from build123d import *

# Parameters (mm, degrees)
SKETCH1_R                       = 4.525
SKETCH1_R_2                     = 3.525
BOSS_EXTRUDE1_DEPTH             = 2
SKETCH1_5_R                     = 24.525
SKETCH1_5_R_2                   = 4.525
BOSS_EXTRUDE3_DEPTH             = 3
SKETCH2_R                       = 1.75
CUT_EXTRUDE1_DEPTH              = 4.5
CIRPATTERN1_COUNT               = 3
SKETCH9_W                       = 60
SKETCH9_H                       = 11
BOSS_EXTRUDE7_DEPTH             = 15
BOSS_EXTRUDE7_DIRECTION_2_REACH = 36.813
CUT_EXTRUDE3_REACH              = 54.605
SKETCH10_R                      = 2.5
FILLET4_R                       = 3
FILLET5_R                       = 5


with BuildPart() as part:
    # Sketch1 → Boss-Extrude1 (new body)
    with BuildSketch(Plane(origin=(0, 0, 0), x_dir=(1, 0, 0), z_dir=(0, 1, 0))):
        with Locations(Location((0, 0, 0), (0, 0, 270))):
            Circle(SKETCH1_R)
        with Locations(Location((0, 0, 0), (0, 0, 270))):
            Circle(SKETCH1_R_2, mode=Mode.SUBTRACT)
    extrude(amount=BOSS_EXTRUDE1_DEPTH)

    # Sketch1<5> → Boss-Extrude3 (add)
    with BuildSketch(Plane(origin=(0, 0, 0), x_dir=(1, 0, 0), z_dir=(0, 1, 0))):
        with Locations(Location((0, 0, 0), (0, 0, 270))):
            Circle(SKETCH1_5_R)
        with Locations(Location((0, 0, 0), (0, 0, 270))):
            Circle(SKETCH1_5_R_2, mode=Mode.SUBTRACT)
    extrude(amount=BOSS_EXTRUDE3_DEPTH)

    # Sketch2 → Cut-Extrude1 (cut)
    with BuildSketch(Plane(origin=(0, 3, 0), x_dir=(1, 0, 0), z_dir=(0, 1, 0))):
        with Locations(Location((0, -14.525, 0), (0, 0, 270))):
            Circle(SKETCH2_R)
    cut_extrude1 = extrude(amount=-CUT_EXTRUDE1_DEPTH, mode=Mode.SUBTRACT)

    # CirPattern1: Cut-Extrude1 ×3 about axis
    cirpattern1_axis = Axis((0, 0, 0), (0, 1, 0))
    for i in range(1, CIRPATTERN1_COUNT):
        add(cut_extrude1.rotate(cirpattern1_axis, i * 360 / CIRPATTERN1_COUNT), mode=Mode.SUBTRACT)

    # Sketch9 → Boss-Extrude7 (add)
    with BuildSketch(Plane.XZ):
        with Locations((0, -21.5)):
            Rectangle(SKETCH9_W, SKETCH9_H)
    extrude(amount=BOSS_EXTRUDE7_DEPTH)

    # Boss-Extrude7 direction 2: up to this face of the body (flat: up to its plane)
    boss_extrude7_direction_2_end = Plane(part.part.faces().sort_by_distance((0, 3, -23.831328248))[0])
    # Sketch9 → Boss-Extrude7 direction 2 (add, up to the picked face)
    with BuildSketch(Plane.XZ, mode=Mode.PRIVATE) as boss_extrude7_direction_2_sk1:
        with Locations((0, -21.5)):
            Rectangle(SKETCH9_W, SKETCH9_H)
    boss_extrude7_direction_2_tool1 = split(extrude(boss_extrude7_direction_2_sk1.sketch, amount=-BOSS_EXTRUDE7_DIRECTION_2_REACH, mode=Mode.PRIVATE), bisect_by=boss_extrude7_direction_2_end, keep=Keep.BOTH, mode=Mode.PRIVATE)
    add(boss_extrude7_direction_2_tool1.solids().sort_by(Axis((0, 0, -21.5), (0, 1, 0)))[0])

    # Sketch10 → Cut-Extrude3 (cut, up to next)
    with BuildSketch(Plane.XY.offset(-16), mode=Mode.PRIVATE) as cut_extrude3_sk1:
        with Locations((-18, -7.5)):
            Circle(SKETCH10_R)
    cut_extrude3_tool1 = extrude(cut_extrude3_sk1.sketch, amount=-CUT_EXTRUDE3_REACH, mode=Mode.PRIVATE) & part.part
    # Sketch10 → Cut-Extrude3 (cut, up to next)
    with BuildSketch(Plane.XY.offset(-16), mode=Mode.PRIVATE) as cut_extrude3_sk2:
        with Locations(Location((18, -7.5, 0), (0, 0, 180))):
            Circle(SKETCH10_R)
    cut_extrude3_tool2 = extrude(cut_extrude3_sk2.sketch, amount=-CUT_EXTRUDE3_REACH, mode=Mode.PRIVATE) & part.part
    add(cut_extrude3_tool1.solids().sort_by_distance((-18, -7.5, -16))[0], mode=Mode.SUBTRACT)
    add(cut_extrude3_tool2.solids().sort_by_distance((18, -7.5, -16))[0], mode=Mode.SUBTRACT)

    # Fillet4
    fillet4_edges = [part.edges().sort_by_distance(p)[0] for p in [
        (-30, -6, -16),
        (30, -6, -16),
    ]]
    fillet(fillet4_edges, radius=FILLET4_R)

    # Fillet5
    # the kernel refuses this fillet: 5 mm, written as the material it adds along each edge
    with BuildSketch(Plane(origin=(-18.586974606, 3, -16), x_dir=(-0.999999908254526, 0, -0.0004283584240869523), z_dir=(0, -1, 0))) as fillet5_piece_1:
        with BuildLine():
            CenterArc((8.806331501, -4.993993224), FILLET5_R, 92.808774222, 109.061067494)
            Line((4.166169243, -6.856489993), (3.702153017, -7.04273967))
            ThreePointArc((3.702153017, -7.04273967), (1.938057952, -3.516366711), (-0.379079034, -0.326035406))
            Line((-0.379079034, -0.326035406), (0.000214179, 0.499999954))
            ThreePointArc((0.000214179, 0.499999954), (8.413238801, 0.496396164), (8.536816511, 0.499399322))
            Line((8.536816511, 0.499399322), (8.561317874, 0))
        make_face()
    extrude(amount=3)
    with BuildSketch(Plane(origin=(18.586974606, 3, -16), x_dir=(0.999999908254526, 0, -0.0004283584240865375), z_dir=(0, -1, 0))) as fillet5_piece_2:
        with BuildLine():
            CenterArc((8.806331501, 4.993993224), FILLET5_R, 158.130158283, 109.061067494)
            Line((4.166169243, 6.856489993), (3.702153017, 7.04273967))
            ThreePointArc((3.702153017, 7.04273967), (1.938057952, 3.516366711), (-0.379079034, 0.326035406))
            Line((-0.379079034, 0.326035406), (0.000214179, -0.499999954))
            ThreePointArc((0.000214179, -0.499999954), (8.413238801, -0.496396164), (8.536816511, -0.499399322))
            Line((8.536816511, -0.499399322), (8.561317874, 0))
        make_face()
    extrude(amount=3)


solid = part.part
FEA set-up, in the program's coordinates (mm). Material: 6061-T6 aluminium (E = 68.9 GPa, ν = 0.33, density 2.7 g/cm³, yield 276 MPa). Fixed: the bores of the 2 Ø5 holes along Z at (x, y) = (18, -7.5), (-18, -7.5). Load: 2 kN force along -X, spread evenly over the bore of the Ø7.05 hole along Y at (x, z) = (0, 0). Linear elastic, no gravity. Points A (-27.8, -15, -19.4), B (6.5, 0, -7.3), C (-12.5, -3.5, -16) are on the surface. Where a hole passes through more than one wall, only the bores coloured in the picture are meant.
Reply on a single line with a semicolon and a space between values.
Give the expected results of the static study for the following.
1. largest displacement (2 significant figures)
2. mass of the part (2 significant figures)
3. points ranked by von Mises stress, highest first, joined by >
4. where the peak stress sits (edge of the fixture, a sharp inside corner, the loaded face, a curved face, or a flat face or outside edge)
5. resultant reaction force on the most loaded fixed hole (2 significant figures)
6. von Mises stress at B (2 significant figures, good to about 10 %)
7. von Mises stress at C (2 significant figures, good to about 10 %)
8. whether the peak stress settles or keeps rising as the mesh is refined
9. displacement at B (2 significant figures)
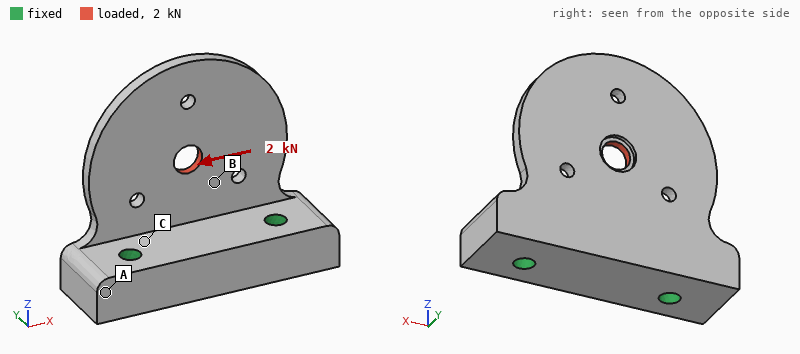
37 µm; 44 g; B > C > A; a sharp inside corner; 1.5 kN; 43 MPa; 18 MPa; keeps rising; 13 µm
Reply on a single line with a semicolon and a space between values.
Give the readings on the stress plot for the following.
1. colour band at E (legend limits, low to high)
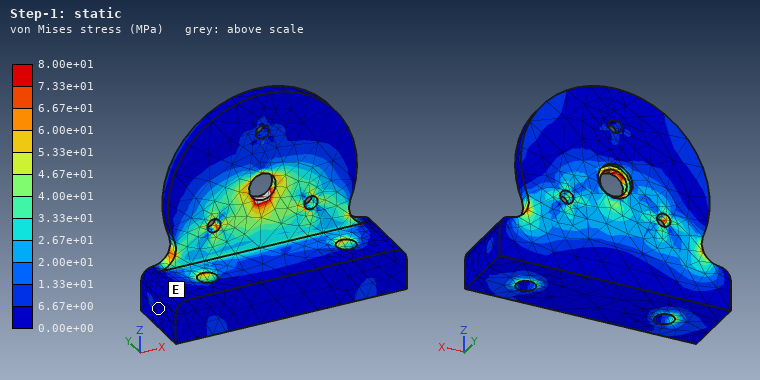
0.00e+00 to 6.67e+00 MPa
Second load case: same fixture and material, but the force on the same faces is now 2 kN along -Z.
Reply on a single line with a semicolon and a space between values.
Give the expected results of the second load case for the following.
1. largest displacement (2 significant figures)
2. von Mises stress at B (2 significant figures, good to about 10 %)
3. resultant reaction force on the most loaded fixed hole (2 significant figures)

58 µm; 35 MPa; 1.0 kN
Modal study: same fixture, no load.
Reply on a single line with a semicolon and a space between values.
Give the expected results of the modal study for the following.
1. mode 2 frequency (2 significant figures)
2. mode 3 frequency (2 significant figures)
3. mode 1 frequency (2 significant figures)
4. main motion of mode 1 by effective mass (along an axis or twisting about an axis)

4000 Hz; 8300 Hz; 1600 Hz; along Y
